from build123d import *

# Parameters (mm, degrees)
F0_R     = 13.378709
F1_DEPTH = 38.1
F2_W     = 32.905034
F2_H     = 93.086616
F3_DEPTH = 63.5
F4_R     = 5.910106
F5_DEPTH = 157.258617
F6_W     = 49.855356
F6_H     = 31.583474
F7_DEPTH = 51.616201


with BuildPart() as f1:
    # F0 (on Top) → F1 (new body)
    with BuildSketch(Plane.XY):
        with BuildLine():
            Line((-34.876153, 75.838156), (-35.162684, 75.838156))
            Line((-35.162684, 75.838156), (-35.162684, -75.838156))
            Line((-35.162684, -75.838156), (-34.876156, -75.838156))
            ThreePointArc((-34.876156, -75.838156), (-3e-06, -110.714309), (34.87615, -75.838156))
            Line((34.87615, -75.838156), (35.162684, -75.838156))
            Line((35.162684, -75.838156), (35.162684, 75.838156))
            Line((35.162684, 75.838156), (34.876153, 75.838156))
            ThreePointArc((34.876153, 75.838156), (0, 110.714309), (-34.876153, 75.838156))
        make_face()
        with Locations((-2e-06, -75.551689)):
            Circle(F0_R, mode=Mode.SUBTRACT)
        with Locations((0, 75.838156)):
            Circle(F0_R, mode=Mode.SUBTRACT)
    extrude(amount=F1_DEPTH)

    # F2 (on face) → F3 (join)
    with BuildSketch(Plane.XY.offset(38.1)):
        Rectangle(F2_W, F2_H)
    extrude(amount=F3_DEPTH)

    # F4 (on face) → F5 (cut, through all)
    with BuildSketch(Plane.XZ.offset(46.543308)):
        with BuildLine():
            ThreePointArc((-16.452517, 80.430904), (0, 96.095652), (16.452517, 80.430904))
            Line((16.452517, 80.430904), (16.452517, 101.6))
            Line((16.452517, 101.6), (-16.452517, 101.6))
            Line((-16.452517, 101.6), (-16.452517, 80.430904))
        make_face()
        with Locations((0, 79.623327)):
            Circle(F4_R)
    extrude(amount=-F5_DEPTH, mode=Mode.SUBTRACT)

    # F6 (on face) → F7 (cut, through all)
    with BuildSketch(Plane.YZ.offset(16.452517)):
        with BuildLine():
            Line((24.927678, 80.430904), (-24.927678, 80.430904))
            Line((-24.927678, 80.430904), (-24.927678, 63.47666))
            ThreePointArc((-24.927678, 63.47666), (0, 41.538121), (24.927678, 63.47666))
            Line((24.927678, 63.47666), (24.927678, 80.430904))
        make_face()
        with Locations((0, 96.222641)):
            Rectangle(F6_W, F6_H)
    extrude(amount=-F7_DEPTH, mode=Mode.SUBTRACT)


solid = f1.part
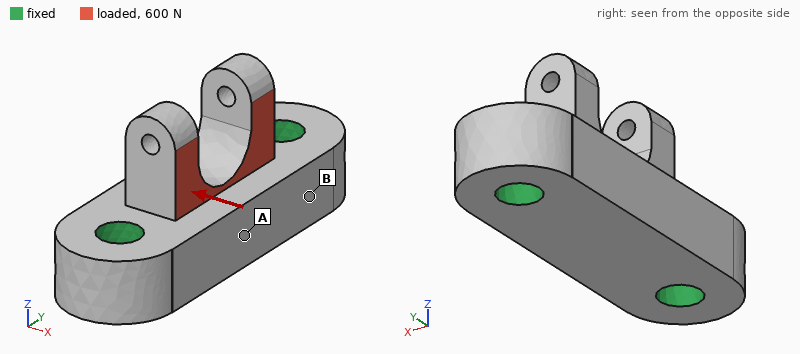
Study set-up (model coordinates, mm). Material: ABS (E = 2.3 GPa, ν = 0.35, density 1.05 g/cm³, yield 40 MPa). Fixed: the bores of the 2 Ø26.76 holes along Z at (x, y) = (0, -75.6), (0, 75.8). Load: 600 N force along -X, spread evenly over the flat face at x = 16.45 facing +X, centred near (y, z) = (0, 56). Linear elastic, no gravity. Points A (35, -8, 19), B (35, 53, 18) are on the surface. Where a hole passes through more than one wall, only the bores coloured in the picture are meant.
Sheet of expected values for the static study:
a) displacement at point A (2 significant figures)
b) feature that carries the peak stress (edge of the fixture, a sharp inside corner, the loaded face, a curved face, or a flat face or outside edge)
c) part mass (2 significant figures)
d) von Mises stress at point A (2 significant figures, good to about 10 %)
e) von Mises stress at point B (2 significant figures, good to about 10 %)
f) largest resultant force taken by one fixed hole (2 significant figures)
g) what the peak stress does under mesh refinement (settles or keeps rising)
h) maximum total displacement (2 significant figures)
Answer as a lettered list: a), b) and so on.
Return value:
a) 20 µm
b) edge of the fixture
c) 630 g
d) 0.20 MPa
e) 0.53 MPa
f) 300 N
g) keeps rising
h) 83 µm
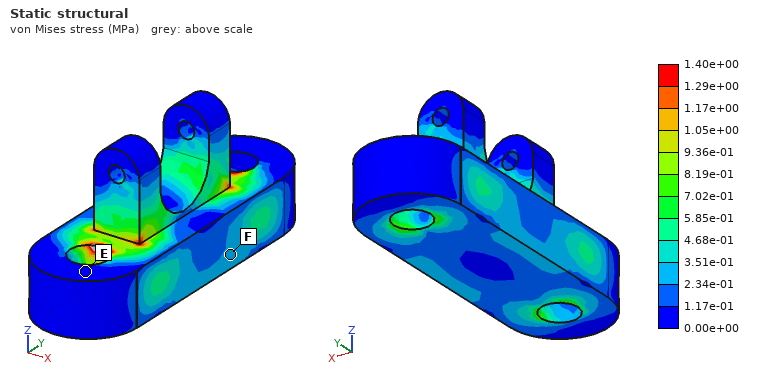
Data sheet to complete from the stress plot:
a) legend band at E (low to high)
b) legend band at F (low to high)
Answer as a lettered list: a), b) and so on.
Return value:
a) 0.00e+00 to 1.17e-01 MPa
b) 2.34e-01 to 3.51e-01 MPa
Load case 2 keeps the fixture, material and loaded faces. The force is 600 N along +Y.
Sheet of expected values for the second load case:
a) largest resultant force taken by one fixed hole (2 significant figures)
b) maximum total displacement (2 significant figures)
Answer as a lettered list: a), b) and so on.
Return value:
a) 350 N
b) 58 µm
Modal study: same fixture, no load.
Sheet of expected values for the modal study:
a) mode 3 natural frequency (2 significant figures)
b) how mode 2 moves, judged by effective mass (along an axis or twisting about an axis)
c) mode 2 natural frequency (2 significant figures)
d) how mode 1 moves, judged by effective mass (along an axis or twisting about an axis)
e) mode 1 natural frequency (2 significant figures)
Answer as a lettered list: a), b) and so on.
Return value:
a) 1900 Hz
b) along Z
c) 1700 Hz
d) along X
e) 1400 Hz
